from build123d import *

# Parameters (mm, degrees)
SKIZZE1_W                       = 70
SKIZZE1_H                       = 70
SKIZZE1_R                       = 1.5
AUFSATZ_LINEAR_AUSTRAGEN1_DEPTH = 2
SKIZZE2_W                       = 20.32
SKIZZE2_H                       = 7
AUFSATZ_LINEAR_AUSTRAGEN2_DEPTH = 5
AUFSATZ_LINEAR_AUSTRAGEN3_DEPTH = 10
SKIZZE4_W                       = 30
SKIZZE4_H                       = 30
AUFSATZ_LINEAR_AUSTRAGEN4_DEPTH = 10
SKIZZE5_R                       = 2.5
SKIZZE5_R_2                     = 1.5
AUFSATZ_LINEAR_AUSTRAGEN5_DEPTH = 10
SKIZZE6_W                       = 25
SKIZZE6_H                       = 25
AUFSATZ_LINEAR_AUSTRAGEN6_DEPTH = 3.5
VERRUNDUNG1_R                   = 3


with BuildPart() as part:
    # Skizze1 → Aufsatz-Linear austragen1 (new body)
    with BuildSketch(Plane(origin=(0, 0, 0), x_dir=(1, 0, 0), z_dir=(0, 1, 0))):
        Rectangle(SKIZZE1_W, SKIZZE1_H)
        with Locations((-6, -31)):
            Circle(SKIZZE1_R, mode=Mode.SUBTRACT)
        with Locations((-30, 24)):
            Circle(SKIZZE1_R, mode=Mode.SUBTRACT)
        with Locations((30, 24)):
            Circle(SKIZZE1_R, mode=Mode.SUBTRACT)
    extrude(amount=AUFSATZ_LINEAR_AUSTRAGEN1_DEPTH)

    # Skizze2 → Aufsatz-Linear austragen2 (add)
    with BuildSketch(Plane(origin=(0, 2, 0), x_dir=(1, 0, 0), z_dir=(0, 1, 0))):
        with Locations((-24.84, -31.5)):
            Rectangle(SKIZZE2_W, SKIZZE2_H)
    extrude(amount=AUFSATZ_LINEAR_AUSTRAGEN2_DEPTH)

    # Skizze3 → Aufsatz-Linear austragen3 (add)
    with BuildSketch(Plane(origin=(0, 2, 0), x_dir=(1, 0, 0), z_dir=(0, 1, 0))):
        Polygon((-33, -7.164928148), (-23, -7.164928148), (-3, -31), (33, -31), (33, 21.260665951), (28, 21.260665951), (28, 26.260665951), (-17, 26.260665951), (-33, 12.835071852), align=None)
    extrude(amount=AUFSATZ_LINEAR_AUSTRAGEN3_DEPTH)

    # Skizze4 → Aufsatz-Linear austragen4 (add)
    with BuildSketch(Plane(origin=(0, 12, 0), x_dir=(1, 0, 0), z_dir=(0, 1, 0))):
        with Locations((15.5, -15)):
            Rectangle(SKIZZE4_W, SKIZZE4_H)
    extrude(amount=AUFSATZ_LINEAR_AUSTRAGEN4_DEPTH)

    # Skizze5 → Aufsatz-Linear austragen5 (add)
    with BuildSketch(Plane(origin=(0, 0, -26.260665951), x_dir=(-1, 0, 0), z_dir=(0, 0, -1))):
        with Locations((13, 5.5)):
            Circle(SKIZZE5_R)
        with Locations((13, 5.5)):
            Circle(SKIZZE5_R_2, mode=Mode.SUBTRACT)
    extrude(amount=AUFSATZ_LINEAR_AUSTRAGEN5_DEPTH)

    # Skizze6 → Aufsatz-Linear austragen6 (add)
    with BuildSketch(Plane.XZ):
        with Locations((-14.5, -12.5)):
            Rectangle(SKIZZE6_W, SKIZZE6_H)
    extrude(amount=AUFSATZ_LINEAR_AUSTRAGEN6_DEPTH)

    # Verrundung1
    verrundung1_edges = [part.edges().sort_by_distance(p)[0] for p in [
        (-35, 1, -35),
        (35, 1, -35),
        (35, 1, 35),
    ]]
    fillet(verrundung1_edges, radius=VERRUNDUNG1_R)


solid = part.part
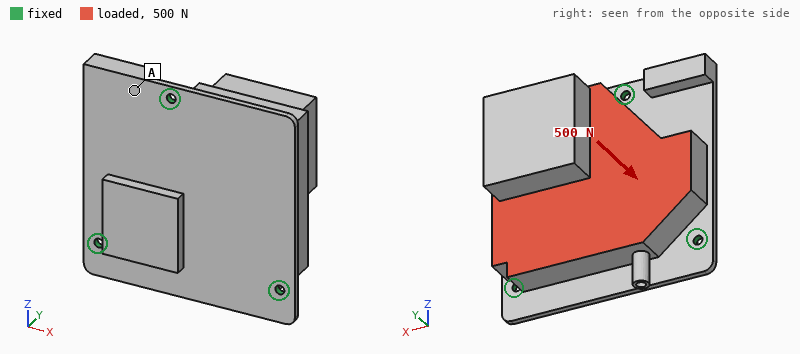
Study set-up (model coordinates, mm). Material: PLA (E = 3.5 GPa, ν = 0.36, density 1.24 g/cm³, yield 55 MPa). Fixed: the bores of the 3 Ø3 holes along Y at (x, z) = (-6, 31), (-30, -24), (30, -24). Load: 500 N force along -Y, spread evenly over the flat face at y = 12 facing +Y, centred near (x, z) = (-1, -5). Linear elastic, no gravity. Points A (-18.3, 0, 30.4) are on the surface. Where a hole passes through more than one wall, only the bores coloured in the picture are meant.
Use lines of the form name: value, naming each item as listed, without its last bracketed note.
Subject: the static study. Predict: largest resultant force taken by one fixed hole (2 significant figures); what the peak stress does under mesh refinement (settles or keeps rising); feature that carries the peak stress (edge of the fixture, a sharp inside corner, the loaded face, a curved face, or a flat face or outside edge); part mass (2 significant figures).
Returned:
largest resultant force taken by one fixed hole: 210 N
what the peak stress does under mesh refinement: keeps rising
feature that carries the peak stress: edge of the fixture
part mass: 66 g
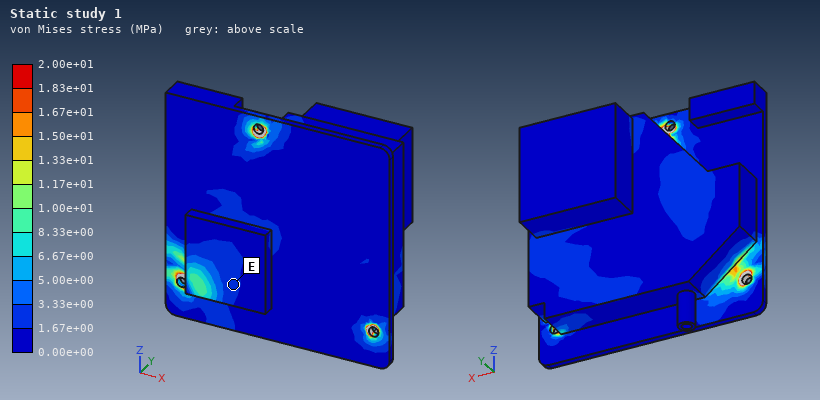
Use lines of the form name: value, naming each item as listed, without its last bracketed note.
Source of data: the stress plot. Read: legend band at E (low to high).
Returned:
legend band at E: 1.67e+00 to 3.33e+00 MPa
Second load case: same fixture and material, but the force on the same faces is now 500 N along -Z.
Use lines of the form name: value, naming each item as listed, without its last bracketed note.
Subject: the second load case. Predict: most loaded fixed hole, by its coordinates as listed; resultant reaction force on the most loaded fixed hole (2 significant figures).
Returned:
most loaded fixed hole, by its coordinates as listed: (-6, 31)
resultant reaction force on the most loaded fixed hole: 240 N
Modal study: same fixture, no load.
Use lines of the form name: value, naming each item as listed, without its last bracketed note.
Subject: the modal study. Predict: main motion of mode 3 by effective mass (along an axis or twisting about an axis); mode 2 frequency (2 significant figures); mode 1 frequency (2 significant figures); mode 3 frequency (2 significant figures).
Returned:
main motion of mode 3 by effective mass: along Y
mode 2 frequency: 1300 Hz
mode 1 frequency: 980 Hz
mode 3 frequency: 1700 Hz
